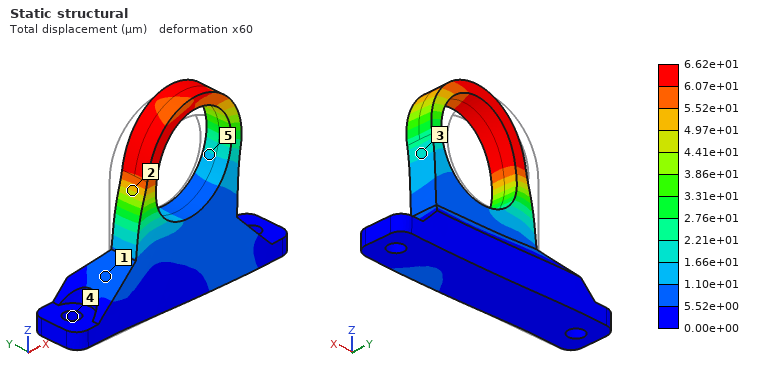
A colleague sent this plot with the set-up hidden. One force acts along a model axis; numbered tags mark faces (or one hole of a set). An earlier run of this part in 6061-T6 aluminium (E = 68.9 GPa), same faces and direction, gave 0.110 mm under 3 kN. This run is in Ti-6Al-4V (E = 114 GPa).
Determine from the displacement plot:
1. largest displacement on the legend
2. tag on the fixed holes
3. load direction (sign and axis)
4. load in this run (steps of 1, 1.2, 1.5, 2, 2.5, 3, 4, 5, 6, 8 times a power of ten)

6.62e+01 µm
4
+X
3 kN
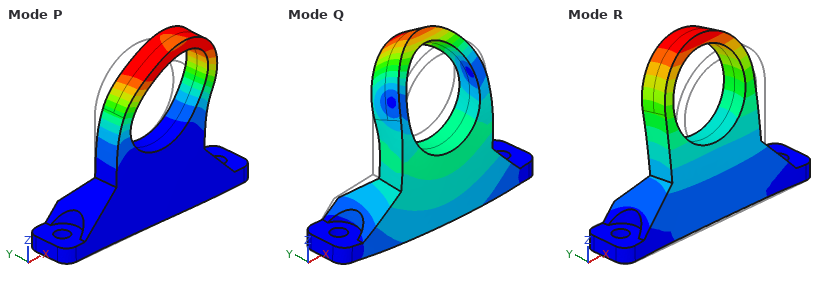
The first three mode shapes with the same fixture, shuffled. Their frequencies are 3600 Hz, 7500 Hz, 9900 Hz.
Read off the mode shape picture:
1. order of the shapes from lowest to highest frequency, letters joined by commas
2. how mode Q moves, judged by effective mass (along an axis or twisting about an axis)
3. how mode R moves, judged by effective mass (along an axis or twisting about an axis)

R, P, Q
along Y
along Y
